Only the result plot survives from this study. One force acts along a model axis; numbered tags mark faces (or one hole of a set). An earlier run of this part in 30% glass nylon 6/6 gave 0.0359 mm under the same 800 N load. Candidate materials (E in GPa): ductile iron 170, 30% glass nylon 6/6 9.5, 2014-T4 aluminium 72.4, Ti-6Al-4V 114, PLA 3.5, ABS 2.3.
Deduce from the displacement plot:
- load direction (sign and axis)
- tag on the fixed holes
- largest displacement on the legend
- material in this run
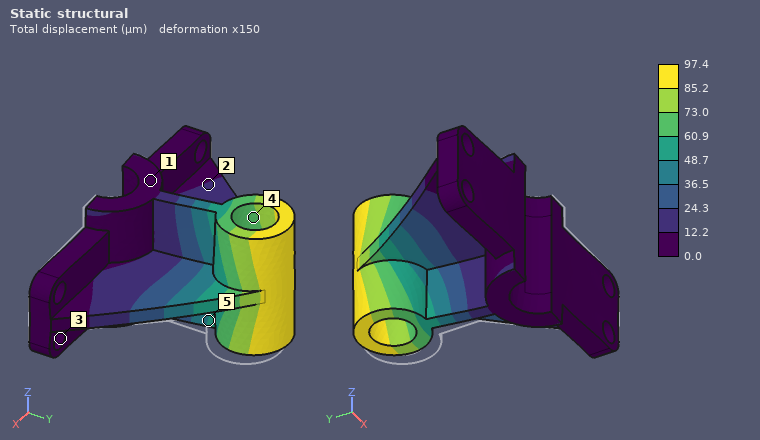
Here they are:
-X
3
97.4 µm
PLA
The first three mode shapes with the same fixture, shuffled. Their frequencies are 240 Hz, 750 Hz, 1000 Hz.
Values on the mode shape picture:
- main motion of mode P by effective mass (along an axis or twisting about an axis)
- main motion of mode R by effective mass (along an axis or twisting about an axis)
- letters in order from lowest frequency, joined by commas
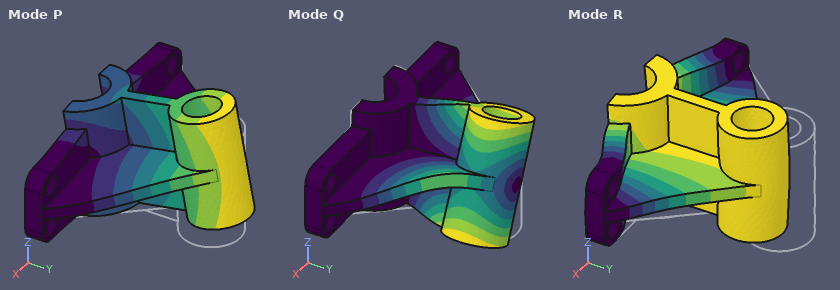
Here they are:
along Z
along Y
P, Q, R
